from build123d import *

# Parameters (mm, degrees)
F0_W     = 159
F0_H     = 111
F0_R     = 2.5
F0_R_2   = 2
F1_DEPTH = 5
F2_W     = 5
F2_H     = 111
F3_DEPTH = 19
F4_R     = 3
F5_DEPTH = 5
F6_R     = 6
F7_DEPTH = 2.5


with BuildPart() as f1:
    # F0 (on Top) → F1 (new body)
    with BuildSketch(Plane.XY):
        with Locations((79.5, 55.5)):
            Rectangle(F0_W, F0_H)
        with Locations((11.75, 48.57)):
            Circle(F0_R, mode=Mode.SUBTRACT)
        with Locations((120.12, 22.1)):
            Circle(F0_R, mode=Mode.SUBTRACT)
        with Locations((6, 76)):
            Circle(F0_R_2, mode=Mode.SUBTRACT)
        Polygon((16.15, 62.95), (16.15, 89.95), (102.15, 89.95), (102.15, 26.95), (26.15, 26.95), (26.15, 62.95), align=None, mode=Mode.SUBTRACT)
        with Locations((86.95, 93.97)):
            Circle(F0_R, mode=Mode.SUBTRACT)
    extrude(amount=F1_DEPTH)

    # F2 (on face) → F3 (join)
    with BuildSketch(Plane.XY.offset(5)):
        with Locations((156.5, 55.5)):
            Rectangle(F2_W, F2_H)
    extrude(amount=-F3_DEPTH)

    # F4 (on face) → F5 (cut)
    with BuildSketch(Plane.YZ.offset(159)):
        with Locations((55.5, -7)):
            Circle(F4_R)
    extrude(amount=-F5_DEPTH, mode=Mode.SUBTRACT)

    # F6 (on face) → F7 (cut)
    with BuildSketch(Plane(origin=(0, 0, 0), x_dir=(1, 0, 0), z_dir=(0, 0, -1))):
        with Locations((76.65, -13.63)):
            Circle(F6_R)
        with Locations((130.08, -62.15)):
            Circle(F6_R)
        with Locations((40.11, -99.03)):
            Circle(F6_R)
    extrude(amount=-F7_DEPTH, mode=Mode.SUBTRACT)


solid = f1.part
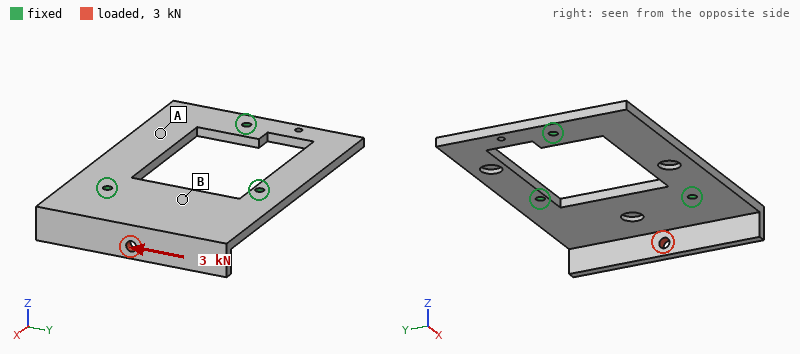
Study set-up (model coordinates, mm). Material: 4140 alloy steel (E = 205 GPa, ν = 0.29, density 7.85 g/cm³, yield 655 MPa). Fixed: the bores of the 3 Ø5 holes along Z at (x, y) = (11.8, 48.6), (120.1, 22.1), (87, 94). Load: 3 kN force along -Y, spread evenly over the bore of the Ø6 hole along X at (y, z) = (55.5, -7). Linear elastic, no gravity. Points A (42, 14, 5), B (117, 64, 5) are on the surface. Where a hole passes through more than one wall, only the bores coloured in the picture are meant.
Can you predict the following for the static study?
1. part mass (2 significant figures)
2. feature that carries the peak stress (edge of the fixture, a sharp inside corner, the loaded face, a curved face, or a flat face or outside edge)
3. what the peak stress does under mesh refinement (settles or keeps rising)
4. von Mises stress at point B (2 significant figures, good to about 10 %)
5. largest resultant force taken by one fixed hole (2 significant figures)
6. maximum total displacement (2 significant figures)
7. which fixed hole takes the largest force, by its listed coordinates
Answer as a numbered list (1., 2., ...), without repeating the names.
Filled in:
1. 540 g
2. edge of the fixture
3. keeps rising
4. 21 MPa
5. 3.2 kN
6. 0.25 mm
7. (120.1, 22.1)
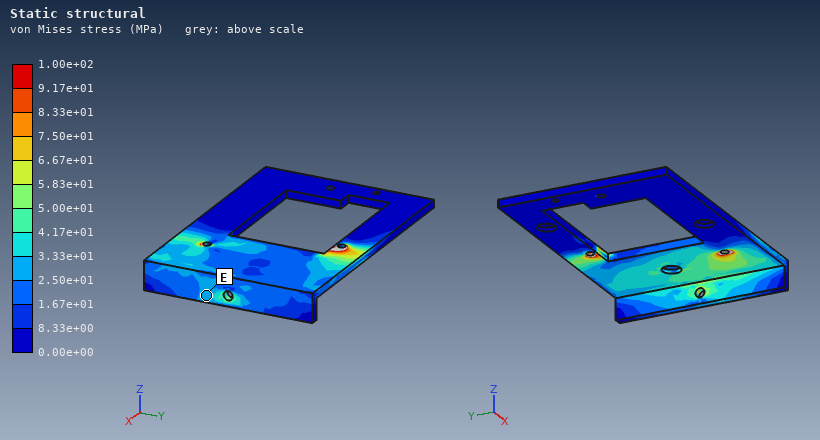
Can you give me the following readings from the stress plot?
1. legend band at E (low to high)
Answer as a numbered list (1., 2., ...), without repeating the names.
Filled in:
1. 2.50e+01 to 3.33e+01 MPa
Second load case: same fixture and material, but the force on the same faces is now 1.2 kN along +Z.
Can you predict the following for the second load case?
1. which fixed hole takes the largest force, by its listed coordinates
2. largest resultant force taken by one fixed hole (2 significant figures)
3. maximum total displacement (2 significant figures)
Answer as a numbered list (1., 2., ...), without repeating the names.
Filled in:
1. (120.1, 22.1)
2. 980 N
3. 0.52 mm
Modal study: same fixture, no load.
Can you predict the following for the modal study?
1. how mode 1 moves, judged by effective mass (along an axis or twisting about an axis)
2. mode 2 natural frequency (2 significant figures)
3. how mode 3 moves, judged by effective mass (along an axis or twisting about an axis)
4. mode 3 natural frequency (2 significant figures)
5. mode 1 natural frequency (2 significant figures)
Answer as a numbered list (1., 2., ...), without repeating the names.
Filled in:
1. along Z
2. 1200 Hz
3. along Z
4. 1400 Hz
5. 760 Hz
